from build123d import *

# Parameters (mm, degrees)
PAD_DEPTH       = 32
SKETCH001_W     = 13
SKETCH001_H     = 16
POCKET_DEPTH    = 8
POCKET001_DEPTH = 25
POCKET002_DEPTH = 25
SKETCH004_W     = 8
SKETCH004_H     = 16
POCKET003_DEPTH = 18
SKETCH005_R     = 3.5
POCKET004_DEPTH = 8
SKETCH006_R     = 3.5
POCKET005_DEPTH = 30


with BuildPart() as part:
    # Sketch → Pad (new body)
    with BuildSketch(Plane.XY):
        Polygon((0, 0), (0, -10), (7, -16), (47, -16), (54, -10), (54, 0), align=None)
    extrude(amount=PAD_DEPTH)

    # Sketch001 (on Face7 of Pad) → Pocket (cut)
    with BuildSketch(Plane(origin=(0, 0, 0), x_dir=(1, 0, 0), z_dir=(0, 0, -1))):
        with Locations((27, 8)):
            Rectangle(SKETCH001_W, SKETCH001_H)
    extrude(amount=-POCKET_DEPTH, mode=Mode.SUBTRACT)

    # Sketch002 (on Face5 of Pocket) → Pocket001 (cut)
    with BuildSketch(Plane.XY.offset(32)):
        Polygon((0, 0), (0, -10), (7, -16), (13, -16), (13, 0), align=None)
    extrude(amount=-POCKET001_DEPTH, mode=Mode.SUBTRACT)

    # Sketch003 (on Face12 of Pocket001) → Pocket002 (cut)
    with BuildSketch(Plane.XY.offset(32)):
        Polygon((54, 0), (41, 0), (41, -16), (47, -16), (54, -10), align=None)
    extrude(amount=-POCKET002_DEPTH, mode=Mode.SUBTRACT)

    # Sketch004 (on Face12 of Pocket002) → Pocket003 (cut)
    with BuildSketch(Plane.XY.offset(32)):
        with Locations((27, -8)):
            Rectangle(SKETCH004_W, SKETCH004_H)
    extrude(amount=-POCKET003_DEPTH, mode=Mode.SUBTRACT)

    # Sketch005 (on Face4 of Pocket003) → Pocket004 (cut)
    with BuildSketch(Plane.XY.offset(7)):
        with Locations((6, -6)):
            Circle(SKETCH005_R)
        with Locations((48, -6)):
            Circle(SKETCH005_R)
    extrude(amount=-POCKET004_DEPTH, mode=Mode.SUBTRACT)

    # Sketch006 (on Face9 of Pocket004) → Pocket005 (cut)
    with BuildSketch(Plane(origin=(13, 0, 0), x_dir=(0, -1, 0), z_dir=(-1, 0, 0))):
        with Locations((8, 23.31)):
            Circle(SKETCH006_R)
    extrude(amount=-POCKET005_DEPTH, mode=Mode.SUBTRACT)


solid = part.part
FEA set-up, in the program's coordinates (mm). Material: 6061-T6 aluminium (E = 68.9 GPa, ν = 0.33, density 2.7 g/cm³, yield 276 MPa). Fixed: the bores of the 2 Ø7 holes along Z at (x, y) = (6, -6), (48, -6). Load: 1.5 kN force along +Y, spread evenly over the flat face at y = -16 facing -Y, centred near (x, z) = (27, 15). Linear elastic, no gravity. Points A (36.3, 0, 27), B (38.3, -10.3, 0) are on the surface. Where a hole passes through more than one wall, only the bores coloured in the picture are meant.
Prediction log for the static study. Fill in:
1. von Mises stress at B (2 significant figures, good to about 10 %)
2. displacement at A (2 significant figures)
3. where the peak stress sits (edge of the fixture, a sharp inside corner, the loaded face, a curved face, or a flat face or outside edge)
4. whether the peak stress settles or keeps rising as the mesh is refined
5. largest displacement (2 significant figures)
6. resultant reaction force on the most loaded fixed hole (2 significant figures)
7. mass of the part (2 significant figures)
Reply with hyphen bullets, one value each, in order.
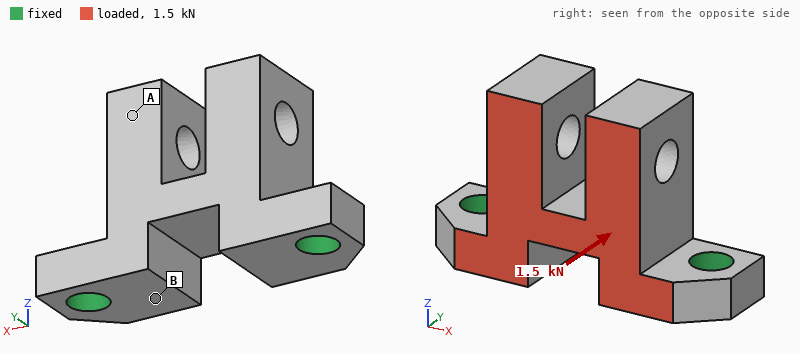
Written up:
- 19 MPa
- 48 µm
- edge of the fixture
- keeps rising
- 59 µm
- 750 N
- 32 g
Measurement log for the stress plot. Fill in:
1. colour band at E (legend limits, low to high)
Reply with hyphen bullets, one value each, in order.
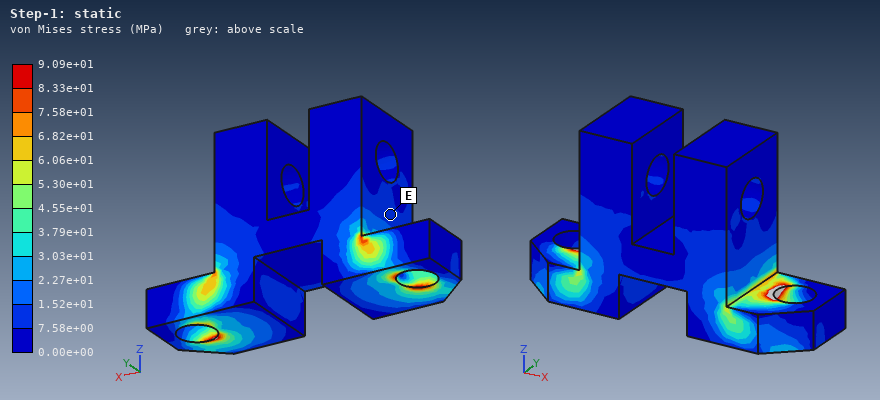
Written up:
- 7.58e+00 to 1.52e+01 MPa
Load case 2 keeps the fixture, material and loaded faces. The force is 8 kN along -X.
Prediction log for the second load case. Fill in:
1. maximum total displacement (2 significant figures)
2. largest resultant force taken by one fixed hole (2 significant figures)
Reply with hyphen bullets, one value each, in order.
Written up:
- 0.12 mm
- 5.1 kN
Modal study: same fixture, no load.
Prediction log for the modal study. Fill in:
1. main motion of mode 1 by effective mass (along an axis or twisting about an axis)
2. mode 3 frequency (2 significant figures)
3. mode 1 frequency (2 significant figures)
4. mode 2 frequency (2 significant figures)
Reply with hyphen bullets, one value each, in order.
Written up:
- along Y
- 11 kHz
- 5900 Hz
- 9800 Hz
